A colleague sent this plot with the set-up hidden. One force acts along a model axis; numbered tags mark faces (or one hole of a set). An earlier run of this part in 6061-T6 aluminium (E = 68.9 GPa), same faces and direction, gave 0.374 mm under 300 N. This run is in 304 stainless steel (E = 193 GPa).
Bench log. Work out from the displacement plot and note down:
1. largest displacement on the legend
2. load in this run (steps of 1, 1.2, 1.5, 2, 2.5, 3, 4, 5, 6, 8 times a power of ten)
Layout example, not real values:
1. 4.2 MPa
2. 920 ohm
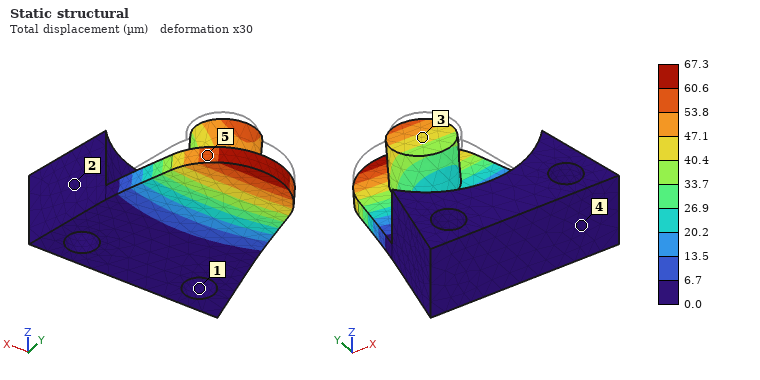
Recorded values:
1. 67.3 µm
2. 150 N
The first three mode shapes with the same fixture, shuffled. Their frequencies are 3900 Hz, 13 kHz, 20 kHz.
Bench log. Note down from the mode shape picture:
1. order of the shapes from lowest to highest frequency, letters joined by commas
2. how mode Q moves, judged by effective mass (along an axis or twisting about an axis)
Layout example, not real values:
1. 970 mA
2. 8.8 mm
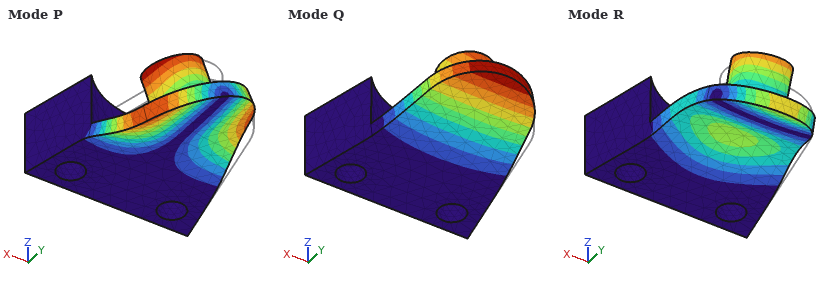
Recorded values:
1. Q, P, R
2. along Z
